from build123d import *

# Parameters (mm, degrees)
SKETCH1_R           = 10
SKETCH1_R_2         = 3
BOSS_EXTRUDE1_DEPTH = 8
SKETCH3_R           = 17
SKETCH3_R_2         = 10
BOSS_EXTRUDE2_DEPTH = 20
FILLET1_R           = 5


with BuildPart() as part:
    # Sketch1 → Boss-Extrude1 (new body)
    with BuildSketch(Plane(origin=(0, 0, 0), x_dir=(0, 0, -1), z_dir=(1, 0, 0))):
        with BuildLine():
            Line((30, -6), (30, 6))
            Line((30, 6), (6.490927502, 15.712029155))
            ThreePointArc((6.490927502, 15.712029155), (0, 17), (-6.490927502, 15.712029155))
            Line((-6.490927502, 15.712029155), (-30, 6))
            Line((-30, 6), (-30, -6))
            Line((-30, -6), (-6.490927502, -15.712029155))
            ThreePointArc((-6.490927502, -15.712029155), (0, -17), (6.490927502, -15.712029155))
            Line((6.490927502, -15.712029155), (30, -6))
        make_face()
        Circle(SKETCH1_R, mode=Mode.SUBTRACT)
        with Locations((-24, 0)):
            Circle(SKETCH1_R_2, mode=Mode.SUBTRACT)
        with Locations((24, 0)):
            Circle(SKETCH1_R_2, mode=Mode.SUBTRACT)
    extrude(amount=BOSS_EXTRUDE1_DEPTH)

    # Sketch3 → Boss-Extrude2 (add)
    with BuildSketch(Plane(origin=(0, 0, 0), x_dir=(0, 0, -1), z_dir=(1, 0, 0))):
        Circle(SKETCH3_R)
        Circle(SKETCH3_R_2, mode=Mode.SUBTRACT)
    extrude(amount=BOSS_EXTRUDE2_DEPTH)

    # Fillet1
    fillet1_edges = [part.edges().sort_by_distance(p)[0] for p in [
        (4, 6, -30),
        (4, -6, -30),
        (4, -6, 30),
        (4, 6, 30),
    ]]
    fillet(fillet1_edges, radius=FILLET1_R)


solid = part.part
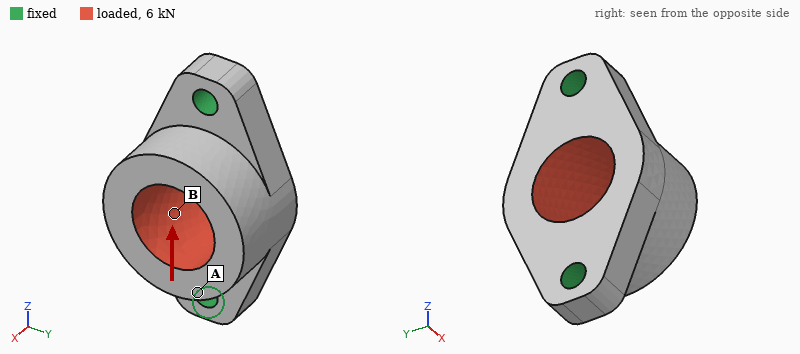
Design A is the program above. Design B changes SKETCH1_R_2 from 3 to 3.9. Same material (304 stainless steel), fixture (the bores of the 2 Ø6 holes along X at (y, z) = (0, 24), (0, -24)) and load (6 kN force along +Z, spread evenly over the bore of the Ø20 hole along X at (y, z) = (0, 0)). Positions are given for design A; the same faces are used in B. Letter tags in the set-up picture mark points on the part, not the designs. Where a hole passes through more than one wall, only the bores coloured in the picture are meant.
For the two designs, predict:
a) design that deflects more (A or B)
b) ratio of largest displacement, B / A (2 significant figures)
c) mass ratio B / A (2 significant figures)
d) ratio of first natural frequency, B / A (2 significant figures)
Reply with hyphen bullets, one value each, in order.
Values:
- A
- 0.91
- 0.98
- 1.1
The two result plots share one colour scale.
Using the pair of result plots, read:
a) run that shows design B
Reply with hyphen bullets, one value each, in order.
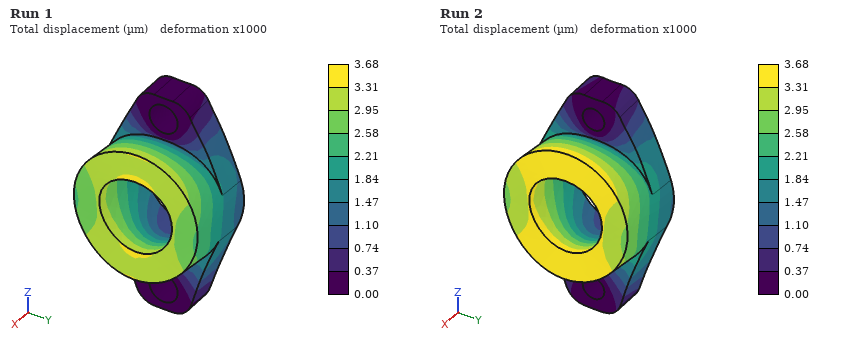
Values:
- Run 1
